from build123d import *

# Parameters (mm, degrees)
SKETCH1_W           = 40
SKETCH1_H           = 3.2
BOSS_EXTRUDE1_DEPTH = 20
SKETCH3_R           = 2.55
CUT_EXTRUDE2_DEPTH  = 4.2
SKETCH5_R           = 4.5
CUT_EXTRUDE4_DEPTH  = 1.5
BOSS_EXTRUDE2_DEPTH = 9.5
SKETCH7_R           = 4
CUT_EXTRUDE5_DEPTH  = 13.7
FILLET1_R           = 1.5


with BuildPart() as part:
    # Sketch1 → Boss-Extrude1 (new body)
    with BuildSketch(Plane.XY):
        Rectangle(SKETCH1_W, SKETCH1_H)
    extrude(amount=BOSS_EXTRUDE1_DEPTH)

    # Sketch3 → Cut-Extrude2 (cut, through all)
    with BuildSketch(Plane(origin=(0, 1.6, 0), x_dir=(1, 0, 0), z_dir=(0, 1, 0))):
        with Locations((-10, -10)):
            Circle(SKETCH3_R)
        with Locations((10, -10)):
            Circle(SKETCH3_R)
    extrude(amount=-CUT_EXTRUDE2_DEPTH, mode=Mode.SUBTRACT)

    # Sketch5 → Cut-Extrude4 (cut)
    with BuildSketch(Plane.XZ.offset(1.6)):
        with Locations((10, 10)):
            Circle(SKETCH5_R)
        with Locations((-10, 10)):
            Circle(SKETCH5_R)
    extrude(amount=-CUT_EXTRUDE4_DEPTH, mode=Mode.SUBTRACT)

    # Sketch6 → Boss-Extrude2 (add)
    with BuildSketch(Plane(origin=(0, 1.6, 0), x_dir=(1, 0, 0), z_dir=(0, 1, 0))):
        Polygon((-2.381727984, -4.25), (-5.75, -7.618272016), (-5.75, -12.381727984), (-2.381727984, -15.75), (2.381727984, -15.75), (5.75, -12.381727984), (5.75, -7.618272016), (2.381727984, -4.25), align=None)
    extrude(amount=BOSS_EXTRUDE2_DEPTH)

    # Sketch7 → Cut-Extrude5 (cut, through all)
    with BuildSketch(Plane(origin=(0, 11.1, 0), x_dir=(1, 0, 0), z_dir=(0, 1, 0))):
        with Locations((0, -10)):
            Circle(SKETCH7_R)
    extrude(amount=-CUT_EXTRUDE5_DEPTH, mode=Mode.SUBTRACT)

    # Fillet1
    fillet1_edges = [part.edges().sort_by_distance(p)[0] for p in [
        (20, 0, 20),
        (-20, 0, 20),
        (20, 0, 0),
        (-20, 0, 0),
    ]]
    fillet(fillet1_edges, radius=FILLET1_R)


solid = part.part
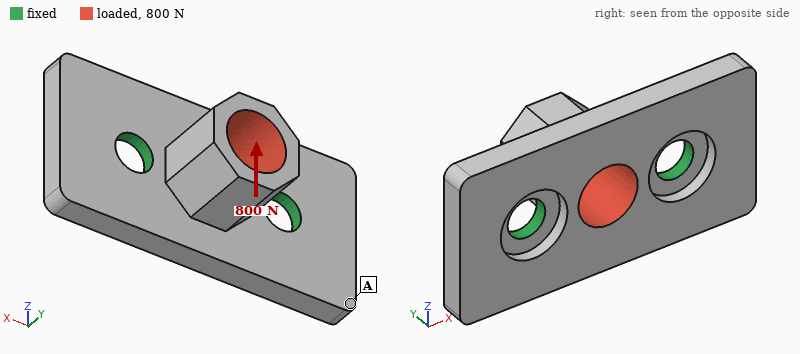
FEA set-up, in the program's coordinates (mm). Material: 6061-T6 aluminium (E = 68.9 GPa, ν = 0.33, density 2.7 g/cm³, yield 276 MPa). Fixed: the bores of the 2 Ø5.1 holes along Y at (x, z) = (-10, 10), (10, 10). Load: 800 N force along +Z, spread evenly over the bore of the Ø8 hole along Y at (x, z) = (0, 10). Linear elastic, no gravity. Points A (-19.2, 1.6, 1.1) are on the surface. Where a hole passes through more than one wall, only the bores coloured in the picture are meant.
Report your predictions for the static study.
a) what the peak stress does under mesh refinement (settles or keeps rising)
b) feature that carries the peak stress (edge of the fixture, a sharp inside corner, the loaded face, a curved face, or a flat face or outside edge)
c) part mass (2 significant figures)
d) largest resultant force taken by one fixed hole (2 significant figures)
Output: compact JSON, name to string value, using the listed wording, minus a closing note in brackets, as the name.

{"what the peak stress does under mesh refinement": "keeps rising", "feature that carries the peak stress": "edge of the fixture", "part mass": "7.3 g", "largest resultant force taken by one fixed hole": "400 N"}
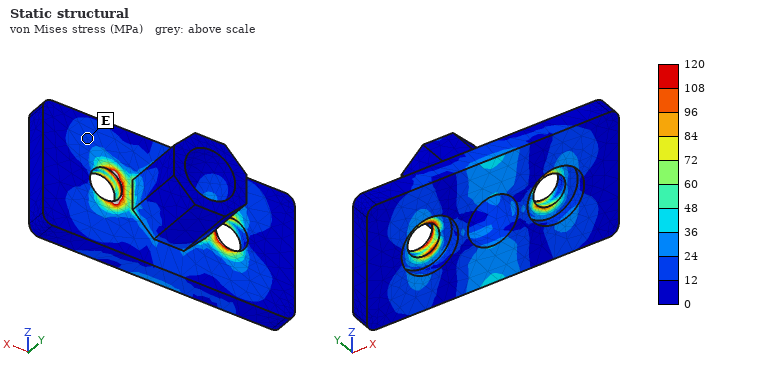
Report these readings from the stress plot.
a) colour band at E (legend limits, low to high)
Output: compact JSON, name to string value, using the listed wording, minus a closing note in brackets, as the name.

{"colour band at E": "12 to 24 MPa"}
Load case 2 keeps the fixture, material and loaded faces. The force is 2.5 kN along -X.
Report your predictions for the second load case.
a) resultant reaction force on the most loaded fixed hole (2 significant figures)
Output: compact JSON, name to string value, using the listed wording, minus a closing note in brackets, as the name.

{"resultant reaction force on the most loaded fixed hole": "1.4 kN"}
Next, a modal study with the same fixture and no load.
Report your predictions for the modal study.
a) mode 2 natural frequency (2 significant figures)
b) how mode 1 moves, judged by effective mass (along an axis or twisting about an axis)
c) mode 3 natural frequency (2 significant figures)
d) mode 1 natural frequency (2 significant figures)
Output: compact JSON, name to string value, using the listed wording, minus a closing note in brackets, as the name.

{"mode 2 natural frequency": "17 kHz", "how mode 1 moves, judged by effective mass": "twisting about X", "mode 3 natural frequency": "18 kHz", "mode 1 natural frequency": "13 kHz"}
